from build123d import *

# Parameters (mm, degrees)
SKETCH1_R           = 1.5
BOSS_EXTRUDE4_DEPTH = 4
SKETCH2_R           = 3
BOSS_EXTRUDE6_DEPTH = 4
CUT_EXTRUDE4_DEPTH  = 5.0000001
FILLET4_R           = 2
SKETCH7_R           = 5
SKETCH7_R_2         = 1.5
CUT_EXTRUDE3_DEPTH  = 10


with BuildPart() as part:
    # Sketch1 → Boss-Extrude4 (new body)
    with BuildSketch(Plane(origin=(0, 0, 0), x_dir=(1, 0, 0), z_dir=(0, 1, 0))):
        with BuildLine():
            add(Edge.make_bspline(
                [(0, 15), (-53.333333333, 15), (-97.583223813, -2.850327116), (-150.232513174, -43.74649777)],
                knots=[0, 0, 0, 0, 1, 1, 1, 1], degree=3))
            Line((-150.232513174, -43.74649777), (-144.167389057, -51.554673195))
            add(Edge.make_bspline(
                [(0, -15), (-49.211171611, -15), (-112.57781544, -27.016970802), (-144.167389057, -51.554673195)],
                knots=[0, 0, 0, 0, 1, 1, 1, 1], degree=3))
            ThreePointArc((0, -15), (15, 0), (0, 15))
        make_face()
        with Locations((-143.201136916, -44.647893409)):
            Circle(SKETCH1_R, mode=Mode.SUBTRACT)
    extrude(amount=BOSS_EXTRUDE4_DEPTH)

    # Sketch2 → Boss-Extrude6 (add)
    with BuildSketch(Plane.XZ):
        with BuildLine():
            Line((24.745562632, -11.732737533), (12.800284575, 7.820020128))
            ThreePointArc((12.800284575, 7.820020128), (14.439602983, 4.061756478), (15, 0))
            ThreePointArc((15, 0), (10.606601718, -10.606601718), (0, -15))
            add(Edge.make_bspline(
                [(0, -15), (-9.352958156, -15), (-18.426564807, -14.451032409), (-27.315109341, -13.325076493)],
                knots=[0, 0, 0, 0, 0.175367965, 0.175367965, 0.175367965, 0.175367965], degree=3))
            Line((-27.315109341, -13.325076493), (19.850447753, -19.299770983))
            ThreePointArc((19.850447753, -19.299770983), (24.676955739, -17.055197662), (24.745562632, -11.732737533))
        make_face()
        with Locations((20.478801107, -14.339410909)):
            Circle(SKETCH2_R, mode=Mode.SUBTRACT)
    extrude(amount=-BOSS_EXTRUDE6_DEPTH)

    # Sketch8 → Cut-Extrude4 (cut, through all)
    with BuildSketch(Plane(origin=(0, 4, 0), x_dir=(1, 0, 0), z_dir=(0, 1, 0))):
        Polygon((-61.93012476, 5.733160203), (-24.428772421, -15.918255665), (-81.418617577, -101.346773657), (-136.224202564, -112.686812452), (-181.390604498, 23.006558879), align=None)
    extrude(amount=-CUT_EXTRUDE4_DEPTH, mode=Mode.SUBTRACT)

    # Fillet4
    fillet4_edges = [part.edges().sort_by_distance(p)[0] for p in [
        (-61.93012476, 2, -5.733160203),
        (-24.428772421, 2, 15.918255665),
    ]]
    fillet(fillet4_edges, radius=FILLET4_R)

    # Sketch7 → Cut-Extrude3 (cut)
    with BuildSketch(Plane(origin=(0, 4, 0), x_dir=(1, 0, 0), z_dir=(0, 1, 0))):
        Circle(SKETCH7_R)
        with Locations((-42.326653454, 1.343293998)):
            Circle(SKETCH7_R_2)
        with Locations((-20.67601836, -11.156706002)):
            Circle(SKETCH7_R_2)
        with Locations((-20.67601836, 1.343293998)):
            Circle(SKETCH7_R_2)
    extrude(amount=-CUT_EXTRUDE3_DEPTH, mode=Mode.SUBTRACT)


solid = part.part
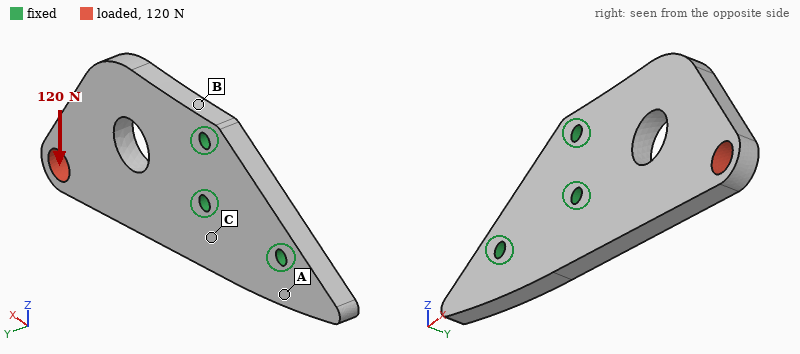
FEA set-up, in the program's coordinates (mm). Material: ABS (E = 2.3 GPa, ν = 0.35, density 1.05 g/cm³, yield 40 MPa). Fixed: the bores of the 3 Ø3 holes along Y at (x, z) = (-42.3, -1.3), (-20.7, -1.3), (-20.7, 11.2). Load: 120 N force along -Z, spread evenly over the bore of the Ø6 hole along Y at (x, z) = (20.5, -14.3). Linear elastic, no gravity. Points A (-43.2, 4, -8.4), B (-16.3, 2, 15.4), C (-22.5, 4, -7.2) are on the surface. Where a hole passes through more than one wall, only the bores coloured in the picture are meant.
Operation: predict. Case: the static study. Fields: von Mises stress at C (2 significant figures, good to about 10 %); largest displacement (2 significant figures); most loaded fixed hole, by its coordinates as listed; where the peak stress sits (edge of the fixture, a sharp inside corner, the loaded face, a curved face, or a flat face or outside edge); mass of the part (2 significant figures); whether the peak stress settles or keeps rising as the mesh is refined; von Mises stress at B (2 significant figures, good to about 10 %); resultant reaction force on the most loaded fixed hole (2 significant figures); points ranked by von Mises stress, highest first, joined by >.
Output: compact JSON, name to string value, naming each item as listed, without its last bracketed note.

{"von Mises stress at C": "3.8 MPa", "largest displacement": "0.40 mm", "most loaded fixed hole, by its coordinates as listed": "(-20.7, 11.2)", "where the peak stress sits": "edge of the fixture", "mass of the part": "7.5 g", "whether the peak stress settles or keeps rising as the mesh is refined": "keeps rising", "von Mises stress at B": "7.6 MPa", "resultant reaction force on the most loaded fixed hole": "260 N", "points ranked by von Mises stress, highest first, joined by >": "B > C > A"}
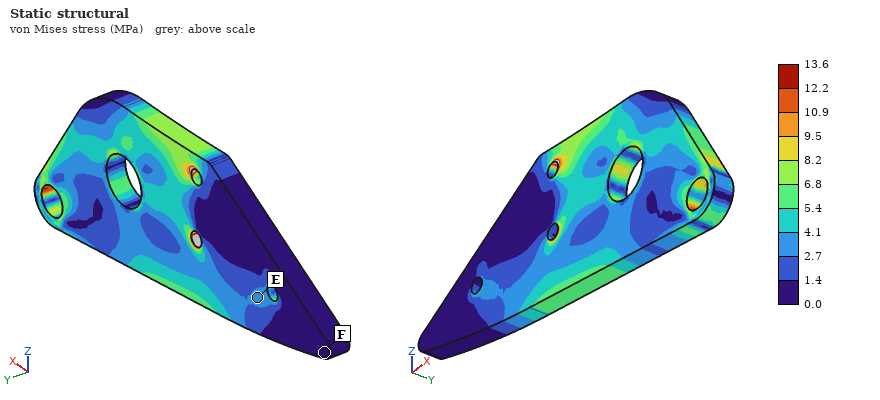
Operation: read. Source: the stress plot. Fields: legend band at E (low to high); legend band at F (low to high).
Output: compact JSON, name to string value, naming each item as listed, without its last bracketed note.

{"legend band at E": "2.7 to 4.1 MPa", "legend band at F": "0.0 to 1.4 MPa"}
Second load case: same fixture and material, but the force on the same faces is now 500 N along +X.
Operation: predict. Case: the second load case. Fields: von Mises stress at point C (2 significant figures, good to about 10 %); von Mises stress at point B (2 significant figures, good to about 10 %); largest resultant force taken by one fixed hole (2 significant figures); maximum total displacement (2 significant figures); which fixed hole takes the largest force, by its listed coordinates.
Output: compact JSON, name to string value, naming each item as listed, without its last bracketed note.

{"von Mises stress at point C": "9.2 MPa", "von Mises stress at point B": "8.6 MPa", "largest resultant force taken by one fixed hole": "550 N", "maximum total displacement": "0.75 mm", "which fixed hole takes the largest force, by its listed coordinates": "(-20.7, -1.3)"}
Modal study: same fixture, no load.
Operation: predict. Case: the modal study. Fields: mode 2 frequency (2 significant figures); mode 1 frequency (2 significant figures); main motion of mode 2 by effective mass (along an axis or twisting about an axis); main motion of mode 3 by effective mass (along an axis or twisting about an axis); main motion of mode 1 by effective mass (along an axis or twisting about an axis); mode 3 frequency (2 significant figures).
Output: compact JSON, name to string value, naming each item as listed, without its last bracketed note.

{"mode 2 frequency": "1700 Hz", "mode 1 frequency": "560 Hz", "main motion of mode 2 by effective mass": "twisting about X", "main motion of mode 3 by effective mass": "along Z", "main motion of mode 1 by effective mass": "along Y", "mode 3 frequency": "2600 Hz"}
